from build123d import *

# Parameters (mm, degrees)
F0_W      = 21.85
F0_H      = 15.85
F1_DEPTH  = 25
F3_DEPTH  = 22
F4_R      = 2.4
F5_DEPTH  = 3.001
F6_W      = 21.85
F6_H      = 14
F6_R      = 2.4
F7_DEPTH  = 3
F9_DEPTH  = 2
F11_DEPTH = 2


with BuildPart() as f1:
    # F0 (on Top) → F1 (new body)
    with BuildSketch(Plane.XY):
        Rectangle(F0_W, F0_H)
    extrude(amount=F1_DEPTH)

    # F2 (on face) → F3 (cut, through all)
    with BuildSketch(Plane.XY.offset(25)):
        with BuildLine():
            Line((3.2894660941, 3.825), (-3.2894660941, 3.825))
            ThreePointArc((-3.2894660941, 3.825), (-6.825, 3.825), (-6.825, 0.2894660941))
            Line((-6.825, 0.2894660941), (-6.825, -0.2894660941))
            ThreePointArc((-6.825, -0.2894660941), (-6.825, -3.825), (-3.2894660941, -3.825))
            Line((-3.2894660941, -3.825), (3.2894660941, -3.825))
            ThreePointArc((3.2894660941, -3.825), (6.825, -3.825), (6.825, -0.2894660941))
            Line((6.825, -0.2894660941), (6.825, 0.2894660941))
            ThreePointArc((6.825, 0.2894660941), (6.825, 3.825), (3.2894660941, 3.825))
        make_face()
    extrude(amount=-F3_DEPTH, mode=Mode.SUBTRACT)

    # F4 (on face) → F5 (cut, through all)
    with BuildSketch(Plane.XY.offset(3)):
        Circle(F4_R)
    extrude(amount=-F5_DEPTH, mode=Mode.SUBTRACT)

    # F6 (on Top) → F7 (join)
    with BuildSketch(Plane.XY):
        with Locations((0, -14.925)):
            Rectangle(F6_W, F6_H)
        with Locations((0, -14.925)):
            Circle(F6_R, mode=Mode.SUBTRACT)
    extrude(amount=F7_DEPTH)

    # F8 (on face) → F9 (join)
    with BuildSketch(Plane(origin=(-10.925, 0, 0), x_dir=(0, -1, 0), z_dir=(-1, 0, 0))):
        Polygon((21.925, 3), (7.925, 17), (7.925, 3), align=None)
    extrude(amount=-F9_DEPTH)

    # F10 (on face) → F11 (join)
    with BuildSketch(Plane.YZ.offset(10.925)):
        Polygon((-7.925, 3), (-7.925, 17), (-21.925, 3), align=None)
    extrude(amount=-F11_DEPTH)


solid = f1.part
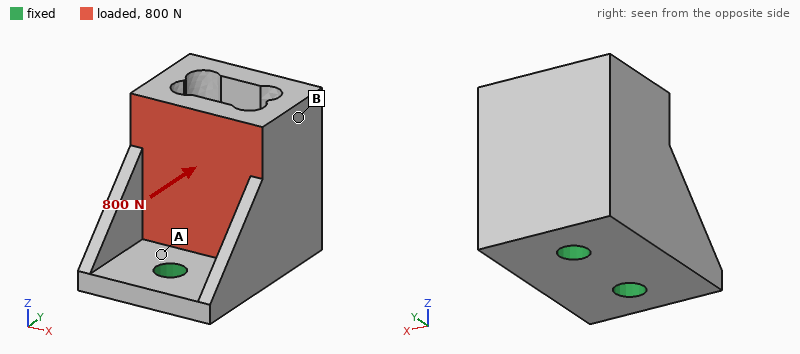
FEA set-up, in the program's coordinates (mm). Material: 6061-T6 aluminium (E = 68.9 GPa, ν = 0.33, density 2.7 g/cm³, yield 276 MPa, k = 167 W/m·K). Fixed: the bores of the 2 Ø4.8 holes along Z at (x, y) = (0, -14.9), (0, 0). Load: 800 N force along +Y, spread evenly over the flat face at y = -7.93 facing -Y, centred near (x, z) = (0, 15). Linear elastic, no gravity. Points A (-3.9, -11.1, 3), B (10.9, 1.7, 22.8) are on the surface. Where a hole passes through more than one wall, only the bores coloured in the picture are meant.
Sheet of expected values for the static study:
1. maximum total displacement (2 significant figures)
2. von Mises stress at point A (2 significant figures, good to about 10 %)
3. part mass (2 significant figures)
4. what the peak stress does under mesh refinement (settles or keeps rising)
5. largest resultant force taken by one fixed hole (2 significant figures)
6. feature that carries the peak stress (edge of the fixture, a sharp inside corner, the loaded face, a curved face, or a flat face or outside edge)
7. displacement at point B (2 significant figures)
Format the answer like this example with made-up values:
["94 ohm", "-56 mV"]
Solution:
["31 µm", "25 MPa", "20 g", "keeps rising", "710 N", "edge of the fixture", "24 µm"]
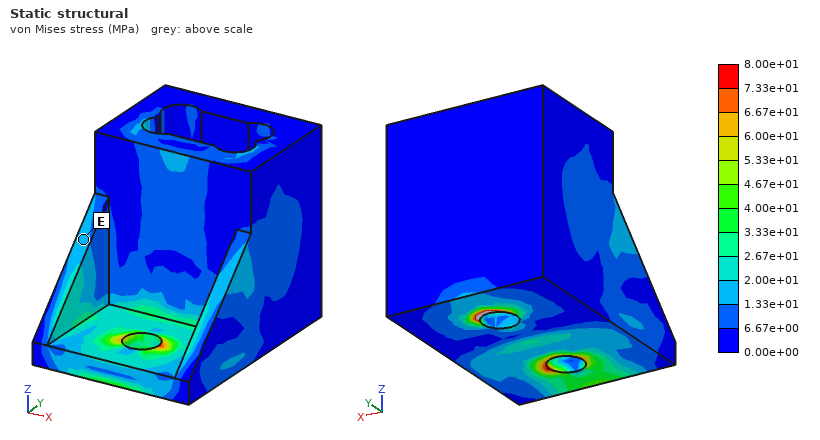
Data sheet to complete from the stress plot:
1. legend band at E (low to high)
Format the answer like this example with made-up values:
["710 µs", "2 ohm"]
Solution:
["1.33e+01 to 2.00e+01 MPa"]
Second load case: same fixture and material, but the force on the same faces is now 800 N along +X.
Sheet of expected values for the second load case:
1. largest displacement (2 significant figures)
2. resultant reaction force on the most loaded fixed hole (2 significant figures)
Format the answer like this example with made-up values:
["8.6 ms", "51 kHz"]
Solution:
["68 µm", "410 N"]
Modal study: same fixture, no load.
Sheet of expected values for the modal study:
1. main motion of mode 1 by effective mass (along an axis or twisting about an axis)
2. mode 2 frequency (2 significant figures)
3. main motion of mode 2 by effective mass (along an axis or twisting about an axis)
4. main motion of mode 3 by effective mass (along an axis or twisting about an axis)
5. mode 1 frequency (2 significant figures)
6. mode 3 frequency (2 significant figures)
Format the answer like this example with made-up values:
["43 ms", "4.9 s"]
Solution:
["along X", "8300 Hz", "along Y", "twisting about Z", "5400 Hz", "19 kHz"]
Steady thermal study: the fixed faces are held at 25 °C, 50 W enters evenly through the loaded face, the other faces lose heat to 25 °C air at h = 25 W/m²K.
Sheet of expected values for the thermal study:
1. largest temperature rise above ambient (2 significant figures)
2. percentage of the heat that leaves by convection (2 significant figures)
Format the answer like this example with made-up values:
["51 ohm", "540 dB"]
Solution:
["33 K", "3.1 %"]
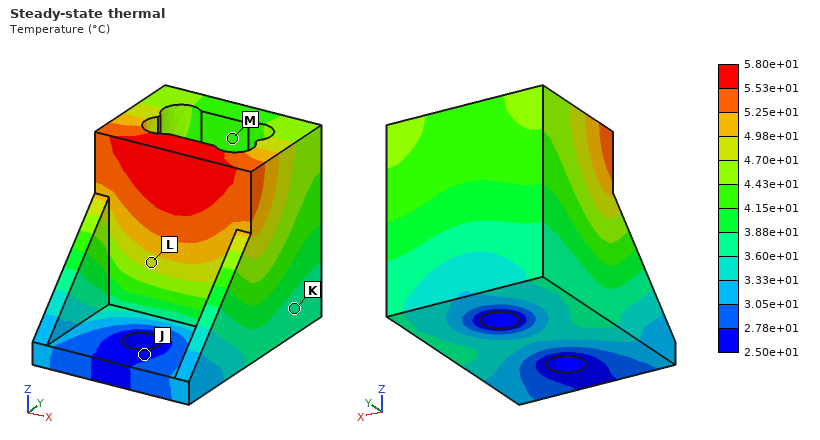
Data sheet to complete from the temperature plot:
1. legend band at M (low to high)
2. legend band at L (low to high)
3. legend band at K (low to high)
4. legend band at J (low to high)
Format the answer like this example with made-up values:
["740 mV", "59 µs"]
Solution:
["4.15e+01 to 4.43e+01 °C", "4.70e+01 to 4.98e+01 °C", "3.60e+01 to 3.88e+01 °C", "2.50e+01 to 2.78e+01 °C"]
